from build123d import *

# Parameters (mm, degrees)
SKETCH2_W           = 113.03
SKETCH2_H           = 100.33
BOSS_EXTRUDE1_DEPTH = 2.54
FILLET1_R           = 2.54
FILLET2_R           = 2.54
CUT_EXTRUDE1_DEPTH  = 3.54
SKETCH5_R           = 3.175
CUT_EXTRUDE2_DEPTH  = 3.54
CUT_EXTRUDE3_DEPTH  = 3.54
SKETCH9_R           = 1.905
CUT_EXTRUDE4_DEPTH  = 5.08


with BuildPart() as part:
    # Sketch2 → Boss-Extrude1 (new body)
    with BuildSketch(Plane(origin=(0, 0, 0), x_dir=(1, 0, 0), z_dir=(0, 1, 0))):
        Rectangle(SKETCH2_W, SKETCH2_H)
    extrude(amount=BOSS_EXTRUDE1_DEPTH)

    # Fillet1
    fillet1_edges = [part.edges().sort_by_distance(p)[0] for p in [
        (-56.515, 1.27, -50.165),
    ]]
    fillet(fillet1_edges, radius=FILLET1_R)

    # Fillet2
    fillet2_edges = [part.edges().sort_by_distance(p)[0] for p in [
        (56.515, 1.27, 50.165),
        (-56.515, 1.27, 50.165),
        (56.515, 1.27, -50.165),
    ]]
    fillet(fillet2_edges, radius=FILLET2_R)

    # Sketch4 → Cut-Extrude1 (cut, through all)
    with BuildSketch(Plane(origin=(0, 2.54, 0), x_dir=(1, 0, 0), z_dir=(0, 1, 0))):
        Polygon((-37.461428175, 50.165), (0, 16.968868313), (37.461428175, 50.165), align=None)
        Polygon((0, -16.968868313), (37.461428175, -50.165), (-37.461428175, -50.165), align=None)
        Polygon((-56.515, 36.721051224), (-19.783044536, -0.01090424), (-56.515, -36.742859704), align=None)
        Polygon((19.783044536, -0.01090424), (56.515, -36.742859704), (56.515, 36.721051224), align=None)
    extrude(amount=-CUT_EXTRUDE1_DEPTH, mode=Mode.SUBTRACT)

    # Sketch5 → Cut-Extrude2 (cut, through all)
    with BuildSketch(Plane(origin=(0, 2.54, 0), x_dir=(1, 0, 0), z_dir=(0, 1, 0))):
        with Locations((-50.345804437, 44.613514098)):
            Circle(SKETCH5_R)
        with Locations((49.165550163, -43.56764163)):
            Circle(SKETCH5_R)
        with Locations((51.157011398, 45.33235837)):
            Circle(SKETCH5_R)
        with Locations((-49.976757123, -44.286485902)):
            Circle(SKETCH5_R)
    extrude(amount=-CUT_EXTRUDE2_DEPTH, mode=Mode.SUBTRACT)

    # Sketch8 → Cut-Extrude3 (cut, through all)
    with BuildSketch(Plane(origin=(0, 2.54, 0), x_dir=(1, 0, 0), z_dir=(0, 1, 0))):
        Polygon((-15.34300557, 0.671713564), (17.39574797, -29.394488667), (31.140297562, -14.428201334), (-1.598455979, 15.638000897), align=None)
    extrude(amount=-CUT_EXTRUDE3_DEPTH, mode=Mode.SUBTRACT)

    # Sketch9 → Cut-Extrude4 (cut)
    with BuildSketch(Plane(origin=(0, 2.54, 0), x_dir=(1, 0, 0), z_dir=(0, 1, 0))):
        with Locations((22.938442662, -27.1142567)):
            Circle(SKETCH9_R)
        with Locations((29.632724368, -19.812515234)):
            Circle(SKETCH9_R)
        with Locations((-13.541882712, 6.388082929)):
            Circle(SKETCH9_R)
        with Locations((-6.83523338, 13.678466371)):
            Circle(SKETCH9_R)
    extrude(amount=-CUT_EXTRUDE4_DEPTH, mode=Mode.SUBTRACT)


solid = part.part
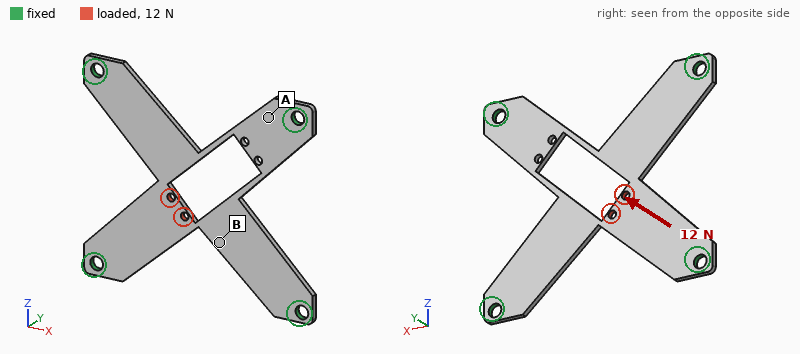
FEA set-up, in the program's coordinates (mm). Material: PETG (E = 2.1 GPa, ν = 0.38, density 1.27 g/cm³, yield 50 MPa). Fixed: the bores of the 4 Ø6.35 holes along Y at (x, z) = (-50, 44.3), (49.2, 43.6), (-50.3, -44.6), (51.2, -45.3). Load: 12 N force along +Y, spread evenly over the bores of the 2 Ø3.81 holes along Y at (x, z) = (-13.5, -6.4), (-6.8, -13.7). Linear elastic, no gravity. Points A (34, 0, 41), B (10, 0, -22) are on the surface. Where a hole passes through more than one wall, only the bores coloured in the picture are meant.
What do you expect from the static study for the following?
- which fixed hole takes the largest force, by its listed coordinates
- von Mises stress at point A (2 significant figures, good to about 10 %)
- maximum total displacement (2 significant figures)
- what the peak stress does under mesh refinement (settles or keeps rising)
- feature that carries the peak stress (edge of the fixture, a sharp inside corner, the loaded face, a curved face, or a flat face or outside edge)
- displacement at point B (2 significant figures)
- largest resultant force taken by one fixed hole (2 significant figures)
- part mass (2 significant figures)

(-50.3, -44.6)
2.3 MPa
1.5 mm
keeps rising
a sharp inside corner
1.1 mm
5.1 N
16 g
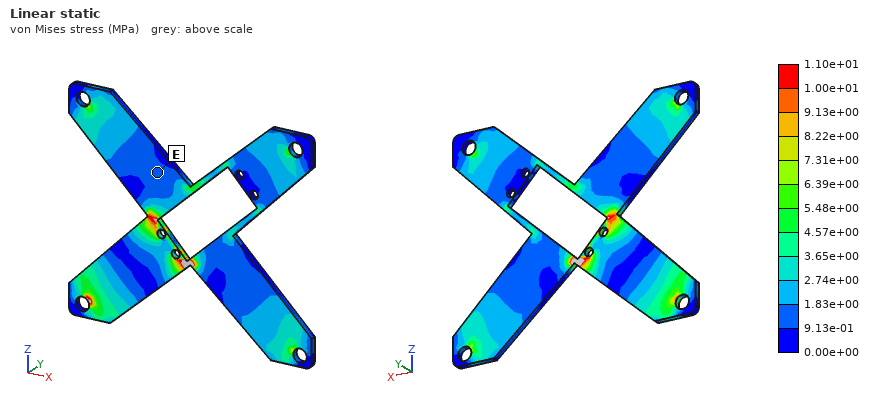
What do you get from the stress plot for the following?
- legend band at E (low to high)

9.13e-01 to 1.83e+00 MPa
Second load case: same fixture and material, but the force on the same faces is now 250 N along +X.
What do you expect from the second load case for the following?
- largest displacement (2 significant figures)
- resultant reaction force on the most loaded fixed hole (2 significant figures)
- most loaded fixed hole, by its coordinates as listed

0.17 mm
140 N
(-50.3, -44.6)
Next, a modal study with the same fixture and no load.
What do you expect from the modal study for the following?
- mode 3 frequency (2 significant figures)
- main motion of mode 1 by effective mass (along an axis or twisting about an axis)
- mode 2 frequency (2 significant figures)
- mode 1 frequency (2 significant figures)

580 Hz
along Y
460 Hz
240 Hz
